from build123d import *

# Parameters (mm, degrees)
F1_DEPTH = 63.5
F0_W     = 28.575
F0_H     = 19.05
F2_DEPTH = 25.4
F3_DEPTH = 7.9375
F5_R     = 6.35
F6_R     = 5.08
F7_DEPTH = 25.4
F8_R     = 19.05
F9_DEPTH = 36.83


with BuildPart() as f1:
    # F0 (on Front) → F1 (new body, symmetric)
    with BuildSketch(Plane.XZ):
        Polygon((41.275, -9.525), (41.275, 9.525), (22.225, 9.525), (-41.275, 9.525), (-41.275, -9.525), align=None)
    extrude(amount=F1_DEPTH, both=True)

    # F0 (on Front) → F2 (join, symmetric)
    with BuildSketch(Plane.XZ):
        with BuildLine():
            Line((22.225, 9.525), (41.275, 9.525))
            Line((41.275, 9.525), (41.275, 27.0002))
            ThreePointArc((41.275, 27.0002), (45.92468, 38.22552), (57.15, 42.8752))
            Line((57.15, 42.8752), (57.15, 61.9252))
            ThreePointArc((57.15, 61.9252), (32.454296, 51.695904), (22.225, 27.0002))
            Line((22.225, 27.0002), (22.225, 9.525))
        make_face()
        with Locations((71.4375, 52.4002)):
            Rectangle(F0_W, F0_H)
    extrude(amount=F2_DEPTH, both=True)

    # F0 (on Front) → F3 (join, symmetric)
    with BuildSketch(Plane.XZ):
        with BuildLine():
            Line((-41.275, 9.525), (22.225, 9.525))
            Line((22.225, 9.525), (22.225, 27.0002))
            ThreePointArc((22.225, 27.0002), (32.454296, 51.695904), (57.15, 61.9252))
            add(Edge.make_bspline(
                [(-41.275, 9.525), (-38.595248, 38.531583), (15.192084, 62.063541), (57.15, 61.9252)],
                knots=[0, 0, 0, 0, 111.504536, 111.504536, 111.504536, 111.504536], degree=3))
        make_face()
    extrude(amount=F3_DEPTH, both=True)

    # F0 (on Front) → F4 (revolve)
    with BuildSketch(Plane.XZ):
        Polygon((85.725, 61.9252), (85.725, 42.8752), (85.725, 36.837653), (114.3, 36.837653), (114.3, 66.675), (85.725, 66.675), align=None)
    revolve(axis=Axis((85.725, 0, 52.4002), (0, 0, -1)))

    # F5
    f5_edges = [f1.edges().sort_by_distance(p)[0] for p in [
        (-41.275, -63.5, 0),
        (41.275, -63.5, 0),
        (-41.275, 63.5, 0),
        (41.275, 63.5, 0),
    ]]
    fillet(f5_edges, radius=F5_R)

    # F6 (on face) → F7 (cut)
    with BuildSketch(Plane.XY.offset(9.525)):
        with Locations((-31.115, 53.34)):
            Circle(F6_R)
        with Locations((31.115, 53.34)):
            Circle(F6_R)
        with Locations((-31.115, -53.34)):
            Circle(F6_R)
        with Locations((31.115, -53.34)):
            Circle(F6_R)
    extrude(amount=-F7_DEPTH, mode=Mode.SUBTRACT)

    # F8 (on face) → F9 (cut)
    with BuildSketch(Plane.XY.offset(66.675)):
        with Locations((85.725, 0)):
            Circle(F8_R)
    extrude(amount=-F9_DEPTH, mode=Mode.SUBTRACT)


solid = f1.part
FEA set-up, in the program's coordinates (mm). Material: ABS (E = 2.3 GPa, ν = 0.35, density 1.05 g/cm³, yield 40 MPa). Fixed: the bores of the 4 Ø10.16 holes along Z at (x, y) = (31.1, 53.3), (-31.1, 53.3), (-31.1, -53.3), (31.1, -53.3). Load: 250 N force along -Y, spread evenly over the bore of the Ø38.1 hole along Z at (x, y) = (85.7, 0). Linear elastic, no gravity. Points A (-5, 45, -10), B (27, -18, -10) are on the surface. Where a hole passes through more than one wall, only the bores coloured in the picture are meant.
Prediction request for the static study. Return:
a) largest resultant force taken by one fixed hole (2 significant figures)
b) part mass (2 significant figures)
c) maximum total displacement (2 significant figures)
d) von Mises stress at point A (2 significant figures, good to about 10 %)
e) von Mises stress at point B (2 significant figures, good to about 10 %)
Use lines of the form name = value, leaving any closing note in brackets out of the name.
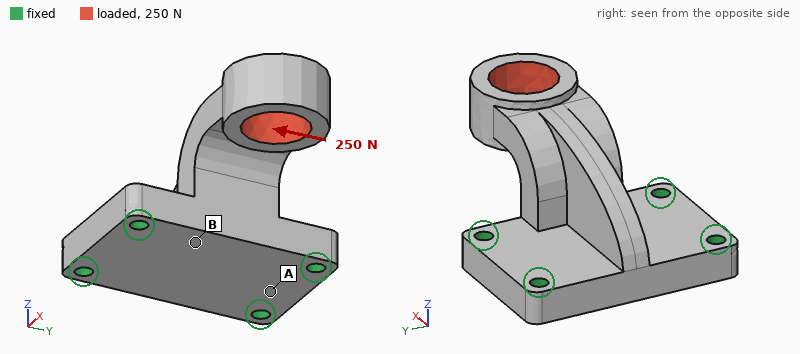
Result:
largest resultant force taken by one fixed hole = 200 N
part mass = 350 g
maximum total displacement = 0.49 mm
von Mises stress at point A = 0.32 MPa
von Mises stress at point B = 0.66 MPa
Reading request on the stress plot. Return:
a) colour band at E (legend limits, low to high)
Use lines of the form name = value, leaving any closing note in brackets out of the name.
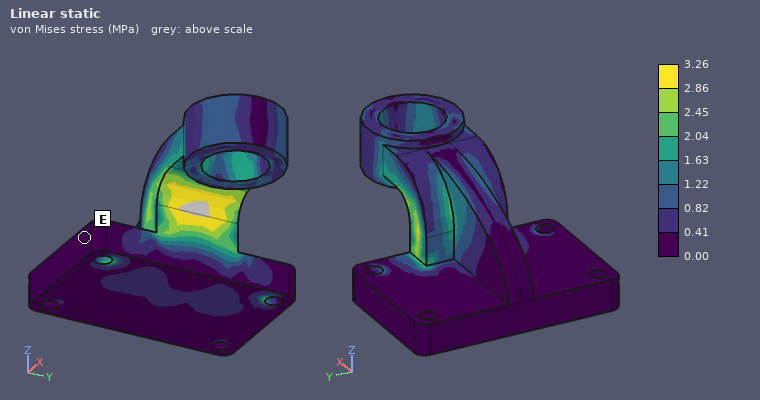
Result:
colour band at E = 0.00 to 0.41 MPa
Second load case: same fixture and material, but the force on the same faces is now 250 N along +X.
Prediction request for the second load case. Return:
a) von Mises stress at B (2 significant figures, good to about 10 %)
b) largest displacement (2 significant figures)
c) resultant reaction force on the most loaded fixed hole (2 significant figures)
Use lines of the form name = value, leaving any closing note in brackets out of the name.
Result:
von Mises stress at B = 0.41 MPa
largest displacement = 0.18 mm
resultant reaction force on the most loaded fixed hole = 140 N
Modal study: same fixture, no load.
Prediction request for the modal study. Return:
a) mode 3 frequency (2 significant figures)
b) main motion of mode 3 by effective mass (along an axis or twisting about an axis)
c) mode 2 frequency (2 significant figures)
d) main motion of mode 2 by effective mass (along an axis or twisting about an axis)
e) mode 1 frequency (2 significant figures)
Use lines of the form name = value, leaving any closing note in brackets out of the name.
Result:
mode 3 frequency = 1200 Hz
main motion of mode 3 by effective mass = along X
mode 2 frequency = 580 Hz
main motion of mode 2 by effective mass = along Y
mode 1 frequency = 520 Hz
